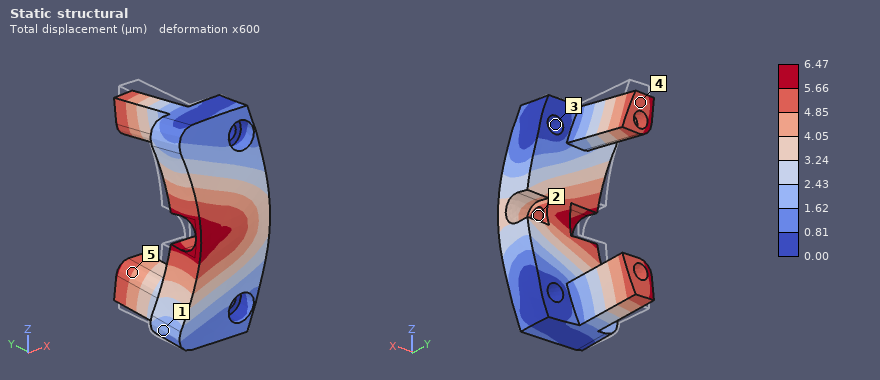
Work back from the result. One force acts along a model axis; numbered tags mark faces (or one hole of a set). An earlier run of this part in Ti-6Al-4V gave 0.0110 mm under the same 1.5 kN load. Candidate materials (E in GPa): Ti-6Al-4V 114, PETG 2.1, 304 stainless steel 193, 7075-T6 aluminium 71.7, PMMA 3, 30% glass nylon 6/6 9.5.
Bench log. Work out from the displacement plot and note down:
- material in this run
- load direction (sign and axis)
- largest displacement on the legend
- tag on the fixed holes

304 stainless steel
-Y
6.47 µm
3
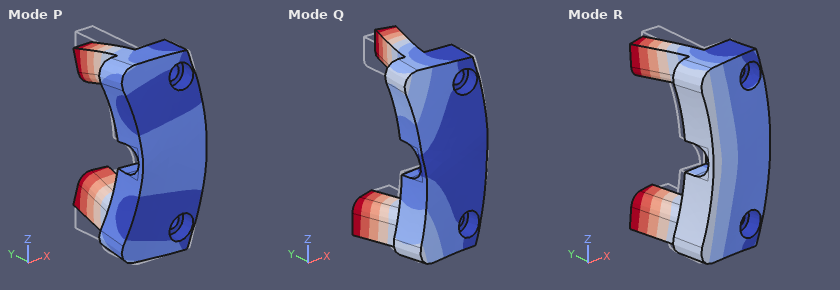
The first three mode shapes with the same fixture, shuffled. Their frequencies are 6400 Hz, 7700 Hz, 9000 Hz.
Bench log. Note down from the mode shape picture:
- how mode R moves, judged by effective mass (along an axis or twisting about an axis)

along Y
